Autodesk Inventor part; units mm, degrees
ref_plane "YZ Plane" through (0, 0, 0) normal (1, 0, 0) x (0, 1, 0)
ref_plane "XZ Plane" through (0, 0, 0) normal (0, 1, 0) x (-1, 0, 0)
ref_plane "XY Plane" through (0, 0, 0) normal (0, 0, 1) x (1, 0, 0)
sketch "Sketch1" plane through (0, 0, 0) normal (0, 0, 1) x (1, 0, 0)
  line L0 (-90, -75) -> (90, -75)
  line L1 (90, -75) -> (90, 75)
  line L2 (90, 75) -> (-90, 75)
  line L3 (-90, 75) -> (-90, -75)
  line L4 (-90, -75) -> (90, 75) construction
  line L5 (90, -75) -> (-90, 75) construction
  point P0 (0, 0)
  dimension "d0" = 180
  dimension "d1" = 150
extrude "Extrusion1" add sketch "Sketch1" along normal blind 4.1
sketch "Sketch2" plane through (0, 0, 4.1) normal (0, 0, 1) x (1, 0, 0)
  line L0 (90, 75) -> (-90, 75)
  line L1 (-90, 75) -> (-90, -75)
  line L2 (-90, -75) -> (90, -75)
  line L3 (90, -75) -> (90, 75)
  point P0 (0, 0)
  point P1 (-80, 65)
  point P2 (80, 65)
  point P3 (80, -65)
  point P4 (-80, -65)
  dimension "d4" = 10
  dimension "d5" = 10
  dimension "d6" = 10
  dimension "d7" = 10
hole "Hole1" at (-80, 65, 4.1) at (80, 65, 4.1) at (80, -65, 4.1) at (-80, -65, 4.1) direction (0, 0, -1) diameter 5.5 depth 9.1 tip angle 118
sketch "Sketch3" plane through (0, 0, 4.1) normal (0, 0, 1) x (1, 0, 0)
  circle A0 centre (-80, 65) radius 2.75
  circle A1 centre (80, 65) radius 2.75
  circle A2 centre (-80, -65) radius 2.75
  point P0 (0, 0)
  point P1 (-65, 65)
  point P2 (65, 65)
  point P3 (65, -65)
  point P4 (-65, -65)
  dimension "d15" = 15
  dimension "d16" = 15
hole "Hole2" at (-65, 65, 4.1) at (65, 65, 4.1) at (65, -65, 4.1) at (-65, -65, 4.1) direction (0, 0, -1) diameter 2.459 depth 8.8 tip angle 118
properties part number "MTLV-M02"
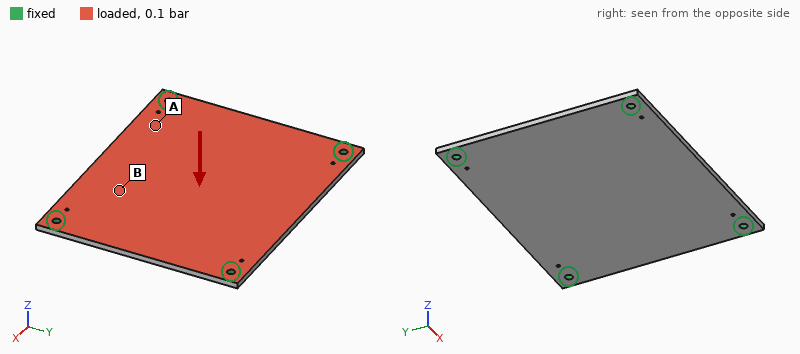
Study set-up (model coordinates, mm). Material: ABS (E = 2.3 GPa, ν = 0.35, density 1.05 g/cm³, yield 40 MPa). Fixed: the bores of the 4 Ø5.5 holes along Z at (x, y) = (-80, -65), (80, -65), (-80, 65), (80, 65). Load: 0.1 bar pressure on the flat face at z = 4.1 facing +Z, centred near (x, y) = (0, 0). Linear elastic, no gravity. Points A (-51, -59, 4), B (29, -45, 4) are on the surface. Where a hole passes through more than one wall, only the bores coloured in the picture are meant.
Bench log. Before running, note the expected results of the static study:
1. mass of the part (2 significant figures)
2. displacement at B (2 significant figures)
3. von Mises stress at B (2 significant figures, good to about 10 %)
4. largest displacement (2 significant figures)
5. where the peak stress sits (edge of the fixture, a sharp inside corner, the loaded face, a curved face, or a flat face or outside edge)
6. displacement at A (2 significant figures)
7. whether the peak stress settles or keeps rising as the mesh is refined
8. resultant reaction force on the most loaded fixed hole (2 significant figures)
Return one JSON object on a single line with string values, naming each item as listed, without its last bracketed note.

{"mass of the part": "120 g", "displacement at B": "1.8 mm", "von Mises stress at B": "3.5 MPa", "largest displacement": "2.6 mm", "where the peak stress sits": "edge of the fixture", "displacement at A": "0.87 mm", "whether the peak stress settles or keeps rising as the mesh is refined": "keeps rising", "resultant reaction force on the most loaded fixed hole": "67 N"}
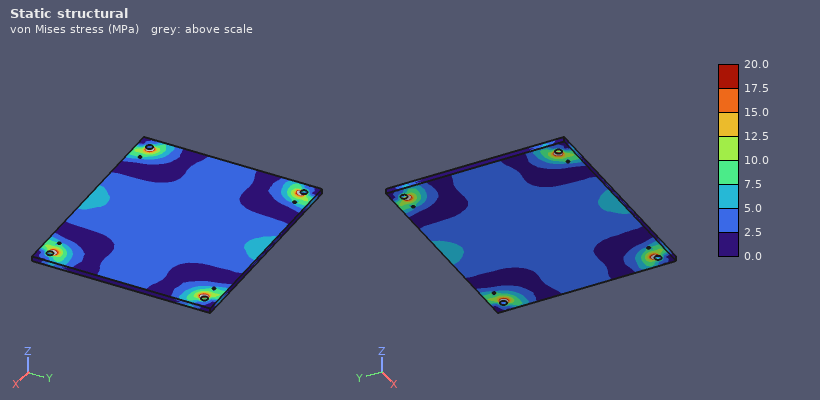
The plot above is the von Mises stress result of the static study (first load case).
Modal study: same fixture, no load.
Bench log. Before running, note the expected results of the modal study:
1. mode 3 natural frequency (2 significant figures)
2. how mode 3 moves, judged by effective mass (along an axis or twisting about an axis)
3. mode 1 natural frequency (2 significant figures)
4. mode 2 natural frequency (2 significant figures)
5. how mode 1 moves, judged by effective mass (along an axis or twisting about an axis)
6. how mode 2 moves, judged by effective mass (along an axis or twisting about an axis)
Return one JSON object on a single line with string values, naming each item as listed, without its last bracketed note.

{"mode 3 natural frequency": "370 Hz", "how mode 3 moves, judged by effective mass": "twisting about Y", "mode 1 natural frequency": "180 Hz", "mode 2 natural frequency": "290 Hz", "how mode 1 moves, judged by effective mass": "along Z", "how mode 2 moves, judged by effective mass": "twisting about X"}
